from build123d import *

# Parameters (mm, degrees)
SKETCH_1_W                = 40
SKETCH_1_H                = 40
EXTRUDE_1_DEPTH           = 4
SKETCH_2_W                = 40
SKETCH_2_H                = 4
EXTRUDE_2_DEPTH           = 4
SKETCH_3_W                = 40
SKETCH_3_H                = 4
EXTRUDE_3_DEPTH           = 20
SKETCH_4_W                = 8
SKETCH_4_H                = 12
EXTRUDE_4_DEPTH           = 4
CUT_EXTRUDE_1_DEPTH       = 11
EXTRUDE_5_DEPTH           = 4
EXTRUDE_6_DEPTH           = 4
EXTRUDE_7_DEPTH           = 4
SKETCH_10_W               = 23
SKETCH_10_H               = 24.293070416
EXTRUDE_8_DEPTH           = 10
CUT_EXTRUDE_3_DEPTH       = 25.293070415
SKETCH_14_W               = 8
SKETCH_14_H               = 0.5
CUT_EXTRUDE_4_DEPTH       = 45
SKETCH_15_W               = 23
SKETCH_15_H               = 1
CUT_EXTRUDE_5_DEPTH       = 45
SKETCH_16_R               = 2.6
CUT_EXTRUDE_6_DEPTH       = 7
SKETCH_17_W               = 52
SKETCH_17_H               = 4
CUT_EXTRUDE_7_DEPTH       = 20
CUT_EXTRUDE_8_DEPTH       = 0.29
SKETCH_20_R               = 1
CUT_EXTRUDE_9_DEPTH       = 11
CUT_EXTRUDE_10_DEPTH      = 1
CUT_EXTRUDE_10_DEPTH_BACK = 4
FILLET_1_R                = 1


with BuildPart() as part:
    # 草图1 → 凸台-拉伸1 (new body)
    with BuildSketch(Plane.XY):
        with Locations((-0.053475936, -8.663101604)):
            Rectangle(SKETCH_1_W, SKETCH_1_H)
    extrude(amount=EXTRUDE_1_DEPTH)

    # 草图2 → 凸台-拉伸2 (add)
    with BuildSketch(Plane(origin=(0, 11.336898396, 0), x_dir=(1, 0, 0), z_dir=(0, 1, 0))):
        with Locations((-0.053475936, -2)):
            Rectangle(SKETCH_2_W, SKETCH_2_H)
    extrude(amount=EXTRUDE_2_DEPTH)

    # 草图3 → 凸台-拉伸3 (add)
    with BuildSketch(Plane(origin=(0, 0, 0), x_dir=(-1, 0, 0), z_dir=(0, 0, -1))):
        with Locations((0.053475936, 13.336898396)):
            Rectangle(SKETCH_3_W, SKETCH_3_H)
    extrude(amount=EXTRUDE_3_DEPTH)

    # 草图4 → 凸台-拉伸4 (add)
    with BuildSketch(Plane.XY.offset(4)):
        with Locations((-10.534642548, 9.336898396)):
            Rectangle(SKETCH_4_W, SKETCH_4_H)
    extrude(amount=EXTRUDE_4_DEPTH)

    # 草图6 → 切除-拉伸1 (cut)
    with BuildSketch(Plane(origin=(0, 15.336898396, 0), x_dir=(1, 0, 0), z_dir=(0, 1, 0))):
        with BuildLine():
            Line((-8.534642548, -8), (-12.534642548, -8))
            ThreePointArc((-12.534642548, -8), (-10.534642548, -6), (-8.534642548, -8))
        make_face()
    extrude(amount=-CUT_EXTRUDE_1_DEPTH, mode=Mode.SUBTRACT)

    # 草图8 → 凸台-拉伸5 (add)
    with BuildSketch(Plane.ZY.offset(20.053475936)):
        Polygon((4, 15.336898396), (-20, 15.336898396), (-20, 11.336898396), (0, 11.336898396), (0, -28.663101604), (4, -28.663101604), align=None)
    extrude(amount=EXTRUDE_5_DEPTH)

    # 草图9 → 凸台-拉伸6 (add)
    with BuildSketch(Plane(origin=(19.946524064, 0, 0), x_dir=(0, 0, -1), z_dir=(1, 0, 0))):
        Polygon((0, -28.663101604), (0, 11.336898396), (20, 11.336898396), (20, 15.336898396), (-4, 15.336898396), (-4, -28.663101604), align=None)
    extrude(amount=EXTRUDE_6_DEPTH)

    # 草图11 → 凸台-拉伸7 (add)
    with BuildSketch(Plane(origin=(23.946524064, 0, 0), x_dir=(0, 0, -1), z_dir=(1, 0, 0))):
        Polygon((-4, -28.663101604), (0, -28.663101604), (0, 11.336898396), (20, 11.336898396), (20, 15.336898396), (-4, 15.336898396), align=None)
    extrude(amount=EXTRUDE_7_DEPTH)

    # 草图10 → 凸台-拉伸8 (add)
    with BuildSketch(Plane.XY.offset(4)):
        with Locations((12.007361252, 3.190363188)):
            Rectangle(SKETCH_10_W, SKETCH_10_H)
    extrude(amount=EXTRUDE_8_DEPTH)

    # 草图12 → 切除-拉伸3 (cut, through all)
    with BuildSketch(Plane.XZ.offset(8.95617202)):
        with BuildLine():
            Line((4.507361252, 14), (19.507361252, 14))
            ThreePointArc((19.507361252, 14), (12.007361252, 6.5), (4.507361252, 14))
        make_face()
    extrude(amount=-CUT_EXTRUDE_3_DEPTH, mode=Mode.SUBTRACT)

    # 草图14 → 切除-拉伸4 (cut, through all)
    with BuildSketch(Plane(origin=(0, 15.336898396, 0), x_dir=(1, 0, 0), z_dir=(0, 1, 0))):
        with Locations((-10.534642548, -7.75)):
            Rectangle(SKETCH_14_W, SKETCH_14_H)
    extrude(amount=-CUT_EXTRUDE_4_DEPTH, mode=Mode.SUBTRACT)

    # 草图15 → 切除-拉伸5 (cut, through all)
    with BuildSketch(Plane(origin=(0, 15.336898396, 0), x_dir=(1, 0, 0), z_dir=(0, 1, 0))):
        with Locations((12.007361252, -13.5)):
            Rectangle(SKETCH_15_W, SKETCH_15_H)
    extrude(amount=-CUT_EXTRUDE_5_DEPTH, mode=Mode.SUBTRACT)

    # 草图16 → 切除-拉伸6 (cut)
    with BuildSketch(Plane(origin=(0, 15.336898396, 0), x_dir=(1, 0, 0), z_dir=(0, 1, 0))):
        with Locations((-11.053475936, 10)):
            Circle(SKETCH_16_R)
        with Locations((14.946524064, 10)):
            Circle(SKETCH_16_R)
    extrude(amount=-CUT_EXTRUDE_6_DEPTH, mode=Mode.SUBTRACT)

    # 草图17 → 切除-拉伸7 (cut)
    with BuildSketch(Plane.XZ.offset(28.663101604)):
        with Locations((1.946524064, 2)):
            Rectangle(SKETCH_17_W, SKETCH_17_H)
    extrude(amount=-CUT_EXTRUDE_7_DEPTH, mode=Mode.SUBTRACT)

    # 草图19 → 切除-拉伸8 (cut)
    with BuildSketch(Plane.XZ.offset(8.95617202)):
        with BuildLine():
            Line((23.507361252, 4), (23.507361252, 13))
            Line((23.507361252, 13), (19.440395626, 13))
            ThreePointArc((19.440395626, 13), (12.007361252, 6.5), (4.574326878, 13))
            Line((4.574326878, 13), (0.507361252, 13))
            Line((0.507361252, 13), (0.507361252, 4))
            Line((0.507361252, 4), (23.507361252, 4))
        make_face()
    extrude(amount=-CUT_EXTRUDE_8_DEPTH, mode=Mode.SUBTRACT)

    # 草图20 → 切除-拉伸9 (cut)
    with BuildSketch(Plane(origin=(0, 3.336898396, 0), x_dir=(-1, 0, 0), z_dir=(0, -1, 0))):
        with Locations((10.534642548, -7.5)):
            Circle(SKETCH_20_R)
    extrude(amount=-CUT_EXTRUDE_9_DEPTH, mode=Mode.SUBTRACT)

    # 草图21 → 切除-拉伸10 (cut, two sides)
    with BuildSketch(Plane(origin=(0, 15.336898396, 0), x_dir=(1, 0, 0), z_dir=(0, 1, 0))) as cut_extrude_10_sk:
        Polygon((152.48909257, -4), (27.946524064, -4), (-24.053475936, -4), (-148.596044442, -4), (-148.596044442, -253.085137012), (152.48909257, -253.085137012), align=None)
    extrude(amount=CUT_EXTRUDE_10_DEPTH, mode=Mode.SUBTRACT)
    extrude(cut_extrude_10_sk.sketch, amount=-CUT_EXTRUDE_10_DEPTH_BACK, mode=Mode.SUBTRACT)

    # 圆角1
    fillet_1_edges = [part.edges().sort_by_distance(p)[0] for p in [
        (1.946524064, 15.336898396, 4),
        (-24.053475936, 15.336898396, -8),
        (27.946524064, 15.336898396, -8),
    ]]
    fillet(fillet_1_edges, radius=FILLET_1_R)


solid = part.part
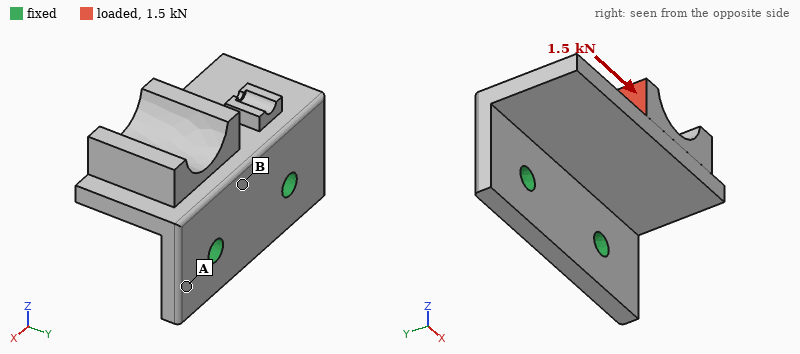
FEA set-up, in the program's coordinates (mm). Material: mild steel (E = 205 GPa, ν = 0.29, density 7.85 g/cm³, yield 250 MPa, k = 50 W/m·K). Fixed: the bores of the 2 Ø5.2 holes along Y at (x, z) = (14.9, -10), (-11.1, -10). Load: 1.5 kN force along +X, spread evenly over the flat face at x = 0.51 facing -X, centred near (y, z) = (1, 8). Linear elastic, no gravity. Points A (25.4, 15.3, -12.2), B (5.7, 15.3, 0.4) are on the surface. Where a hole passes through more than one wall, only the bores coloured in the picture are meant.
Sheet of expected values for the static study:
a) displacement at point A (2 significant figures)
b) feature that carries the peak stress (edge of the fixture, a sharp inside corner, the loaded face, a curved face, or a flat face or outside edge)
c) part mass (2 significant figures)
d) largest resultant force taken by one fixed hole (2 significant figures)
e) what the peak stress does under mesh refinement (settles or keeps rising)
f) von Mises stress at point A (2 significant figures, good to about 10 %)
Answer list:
2.6 µm
edge of the fixture
93 g
1.3 kN
keeps rising
25 MPa
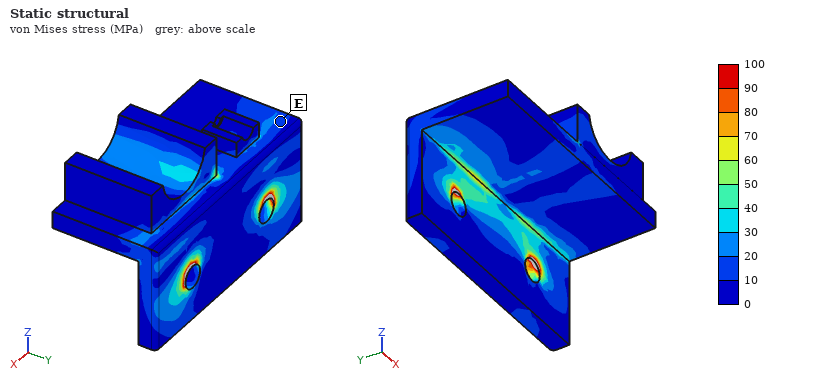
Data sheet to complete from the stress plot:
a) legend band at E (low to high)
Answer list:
10 to 20 MPa
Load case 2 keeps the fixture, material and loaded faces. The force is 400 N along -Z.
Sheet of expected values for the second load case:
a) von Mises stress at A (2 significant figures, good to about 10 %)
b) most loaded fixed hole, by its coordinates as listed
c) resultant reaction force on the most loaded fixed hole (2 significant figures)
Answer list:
9.4 MPa
(-11.1, -10)
230 N
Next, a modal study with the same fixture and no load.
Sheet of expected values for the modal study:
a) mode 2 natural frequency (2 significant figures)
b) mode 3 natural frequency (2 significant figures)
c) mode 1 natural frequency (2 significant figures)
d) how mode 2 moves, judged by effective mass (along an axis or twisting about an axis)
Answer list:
6000 Hz
9300 Hz
2700 Hz
along X
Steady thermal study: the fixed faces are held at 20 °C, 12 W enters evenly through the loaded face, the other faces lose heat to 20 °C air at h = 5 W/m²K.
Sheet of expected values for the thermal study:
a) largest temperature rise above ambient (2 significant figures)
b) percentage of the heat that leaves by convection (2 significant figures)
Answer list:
40 K
3.6 %
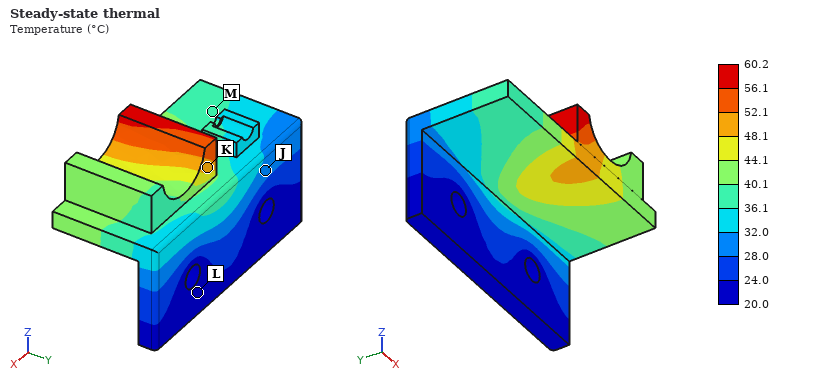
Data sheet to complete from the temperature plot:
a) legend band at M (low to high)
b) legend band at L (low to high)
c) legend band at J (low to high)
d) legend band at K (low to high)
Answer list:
36.1 to 40.1 °C
20.0 to 24.0 °C
28.0 to 32.0 °C
48.1 to 52.1 °C
